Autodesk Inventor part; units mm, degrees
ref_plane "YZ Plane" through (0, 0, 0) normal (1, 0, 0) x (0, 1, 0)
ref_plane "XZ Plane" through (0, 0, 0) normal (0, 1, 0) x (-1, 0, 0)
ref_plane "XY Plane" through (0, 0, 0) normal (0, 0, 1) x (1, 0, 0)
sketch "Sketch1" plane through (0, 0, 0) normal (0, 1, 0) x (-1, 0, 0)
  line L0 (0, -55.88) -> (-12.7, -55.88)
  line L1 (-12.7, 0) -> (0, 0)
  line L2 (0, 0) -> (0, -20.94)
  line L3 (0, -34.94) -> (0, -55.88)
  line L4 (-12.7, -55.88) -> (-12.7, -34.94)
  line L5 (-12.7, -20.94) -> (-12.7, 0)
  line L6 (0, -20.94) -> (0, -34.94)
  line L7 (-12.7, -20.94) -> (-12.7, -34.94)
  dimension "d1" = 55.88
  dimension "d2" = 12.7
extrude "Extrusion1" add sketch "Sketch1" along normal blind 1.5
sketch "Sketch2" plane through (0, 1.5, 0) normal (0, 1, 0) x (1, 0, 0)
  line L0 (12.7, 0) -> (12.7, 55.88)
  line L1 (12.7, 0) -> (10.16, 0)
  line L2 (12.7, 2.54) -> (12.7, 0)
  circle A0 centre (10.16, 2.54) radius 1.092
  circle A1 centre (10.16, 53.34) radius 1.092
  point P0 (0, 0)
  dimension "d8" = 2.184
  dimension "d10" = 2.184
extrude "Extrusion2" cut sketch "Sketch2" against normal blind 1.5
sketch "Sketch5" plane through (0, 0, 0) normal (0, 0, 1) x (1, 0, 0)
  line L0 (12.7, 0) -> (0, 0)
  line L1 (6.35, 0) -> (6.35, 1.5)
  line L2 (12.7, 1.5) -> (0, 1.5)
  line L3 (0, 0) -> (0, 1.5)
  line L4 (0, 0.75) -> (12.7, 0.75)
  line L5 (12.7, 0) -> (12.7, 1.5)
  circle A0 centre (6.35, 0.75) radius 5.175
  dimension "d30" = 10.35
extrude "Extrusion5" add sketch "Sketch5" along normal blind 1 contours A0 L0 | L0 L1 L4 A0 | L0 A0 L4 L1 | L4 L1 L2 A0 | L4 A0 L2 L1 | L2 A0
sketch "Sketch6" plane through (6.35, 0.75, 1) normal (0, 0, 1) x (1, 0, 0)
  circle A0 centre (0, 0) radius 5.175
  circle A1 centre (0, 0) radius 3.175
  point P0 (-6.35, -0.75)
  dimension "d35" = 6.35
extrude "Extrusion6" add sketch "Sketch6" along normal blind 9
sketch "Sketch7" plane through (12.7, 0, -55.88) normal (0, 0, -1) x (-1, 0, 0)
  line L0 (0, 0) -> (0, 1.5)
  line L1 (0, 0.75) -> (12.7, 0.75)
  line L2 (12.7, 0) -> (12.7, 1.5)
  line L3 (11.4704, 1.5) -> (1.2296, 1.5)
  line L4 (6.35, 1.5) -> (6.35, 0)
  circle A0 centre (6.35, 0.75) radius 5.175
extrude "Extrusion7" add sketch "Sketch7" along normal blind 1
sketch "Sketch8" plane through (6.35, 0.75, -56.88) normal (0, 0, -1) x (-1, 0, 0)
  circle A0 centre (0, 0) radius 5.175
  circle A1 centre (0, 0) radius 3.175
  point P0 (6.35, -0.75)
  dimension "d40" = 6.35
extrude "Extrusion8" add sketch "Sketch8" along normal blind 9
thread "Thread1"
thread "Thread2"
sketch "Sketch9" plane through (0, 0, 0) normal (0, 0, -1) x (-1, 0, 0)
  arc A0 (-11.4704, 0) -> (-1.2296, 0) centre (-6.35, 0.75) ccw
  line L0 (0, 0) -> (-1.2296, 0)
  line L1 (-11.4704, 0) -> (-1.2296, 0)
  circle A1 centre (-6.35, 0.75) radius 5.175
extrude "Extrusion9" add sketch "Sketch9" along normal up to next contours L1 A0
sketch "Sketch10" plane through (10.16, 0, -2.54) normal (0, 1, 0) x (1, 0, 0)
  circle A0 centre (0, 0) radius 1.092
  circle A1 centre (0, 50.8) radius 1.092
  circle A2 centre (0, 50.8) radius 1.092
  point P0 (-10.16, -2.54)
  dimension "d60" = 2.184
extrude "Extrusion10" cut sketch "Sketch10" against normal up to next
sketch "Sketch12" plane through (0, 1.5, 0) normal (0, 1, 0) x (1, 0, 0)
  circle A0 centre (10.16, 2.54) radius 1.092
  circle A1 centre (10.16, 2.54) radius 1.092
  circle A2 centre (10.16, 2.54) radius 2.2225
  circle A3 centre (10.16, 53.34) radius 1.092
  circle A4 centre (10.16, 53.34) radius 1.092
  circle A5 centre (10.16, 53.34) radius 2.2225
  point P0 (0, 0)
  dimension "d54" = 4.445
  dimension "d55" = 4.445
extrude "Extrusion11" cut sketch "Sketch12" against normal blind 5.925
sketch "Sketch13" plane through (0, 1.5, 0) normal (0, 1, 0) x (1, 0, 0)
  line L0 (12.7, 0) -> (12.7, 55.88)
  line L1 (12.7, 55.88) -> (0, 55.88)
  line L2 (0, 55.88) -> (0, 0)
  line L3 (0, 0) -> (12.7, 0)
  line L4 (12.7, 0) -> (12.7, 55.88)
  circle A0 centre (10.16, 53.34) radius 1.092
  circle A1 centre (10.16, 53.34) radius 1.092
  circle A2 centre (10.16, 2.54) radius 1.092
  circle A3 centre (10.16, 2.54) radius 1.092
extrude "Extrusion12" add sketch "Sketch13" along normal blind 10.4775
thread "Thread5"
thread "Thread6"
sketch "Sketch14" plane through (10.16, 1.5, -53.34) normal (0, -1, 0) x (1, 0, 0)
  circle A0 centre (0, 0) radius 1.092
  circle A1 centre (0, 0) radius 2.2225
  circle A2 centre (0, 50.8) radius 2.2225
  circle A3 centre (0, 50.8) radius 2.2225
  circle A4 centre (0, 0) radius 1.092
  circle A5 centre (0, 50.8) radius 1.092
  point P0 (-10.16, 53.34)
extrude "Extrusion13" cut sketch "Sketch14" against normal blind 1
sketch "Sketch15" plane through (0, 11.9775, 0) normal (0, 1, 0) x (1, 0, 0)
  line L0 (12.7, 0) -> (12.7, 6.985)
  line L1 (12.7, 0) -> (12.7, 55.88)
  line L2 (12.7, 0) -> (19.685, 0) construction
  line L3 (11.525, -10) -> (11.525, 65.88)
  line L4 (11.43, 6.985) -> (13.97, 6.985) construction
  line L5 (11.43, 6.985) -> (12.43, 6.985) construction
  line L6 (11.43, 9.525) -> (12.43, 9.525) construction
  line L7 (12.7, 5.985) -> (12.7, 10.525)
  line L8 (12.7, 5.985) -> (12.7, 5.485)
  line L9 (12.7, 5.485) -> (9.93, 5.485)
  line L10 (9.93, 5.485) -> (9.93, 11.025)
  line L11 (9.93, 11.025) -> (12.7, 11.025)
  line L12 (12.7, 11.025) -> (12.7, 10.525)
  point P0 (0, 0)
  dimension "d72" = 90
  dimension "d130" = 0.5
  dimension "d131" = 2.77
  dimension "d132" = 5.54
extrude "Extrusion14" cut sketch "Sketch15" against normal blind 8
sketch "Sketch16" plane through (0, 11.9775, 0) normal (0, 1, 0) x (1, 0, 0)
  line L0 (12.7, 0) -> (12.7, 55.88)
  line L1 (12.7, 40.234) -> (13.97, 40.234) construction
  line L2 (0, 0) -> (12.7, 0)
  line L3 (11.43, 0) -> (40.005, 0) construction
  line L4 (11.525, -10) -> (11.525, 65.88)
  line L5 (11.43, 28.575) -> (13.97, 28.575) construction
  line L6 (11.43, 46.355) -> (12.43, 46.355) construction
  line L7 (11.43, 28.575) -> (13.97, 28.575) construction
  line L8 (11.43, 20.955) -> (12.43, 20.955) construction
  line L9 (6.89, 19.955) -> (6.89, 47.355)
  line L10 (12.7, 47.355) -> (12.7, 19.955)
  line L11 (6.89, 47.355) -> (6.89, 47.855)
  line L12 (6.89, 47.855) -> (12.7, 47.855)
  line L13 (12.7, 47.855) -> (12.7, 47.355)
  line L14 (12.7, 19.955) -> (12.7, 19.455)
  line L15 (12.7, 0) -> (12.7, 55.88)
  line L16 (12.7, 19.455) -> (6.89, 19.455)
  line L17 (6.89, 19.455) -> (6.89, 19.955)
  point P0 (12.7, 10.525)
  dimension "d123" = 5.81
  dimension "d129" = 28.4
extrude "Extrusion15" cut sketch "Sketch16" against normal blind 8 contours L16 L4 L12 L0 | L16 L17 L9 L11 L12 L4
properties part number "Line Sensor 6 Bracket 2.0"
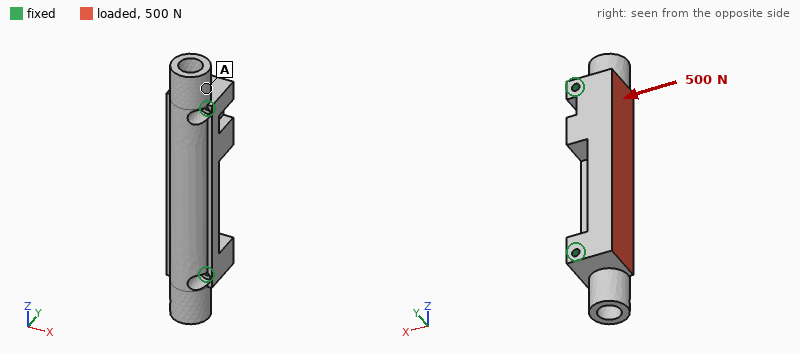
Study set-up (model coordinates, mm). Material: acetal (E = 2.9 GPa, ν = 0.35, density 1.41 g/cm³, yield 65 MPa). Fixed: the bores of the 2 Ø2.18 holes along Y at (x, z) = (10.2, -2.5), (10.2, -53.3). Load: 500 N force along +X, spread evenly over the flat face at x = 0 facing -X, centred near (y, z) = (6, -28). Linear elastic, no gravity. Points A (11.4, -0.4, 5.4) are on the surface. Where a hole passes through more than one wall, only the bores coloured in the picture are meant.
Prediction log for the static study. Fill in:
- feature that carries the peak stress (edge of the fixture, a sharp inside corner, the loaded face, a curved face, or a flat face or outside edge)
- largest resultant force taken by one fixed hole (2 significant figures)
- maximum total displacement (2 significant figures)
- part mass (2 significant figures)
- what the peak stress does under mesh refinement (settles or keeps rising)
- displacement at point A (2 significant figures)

edge of the fixture
330 N
0.12 mm
14 g
keeps rising
0.022 mm
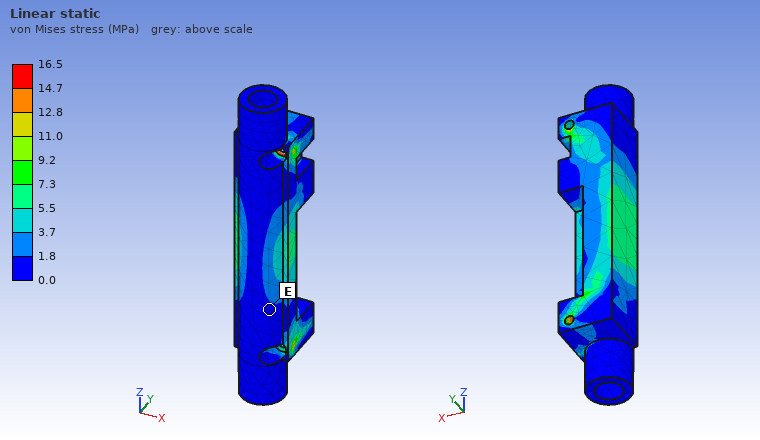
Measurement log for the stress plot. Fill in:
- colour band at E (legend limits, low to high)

0.0 to 1.8 MPa
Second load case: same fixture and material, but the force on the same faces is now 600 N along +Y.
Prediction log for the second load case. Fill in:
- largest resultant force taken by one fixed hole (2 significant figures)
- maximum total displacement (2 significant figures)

320 N
0.21 mm
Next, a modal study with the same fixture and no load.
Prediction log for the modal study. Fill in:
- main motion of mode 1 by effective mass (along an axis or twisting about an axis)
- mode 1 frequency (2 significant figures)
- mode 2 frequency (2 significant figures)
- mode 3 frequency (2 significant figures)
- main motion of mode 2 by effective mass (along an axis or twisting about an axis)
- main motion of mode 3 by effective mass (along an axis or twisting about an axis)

along X
3400 Hz
3900 Hz
5100 Hz
along Y
twisting about Z
